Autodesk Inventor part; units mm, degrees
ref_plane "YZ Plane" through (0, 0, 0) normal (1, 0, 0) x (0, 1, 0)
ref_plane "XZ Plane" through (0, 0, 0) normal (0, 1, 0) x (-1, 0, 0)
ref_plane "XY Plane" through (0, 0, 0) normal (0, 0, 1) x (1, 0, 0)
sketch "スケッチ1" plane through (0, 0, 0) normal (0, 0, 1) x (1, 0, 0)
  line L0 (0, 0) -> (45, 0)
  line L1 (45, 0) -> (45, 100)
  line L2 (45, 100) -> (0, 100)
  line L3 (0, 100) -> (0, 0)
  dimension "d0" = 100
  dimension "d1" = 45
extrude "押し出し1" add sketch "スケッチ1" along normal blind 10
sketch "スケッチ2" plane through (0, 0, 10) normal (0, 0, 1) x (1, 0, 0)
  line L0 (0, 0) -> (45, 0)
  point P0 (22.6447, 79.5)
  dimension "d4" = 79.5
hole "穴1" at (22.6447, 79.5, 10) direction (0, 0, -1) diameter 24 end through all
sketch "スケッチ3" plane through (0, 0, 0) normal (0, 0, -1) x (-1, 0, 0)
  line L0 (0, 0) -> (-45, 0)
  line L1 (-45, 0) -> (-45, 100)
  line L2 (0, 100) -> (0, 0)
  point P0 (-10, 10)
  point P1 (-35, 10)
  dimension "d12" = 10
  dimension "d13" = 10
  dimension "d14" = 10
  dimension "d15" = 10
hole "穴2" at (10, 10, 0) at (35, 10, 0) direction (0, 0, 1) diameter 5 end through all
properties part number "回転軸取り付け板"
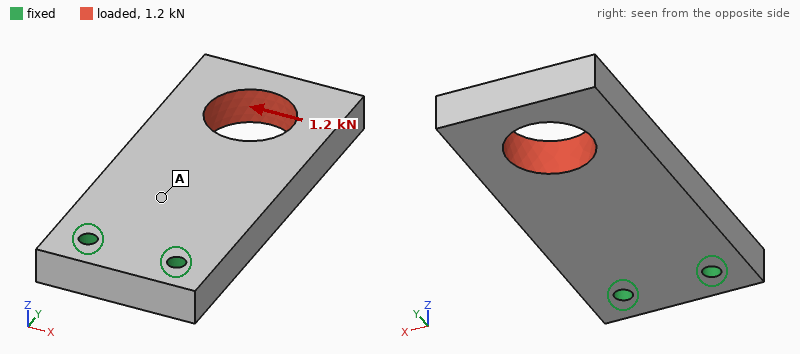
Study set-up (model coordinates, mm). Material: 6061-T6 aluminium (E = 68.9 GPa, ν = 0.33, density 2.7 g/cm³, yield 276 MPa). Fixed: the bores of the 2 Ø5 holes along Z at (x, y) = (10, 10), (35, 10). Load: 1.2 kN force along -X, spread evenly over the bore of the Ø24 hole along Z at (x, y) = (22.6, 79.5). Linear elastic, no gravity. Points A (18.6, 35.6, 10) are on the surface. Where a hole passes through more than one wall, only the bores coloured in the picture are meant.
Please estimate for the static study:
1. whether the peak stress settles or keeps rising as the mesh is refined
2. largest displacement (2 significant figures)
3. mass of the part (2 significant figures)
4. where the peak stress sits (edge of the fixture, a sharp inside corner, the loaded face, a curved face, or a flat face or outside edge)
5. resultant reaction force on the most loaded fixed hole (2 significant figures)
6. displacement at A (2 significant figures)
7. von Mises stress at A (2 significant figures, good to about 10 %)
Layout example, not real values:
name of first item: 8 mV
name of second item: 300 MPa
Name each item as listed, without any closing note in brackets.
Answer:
whether the peak stress settles or keeps rising as the mesh is refined: keeps rising
largest displacement: 63 µm
mass of the part: 110 g
where the peak stress sits: edge of the fixture
resultant reaction force on the most loaded fixed hole: 3.0 kN
displacement at A: 9.8 µm
von Mises stress at A: 7.9 MPa
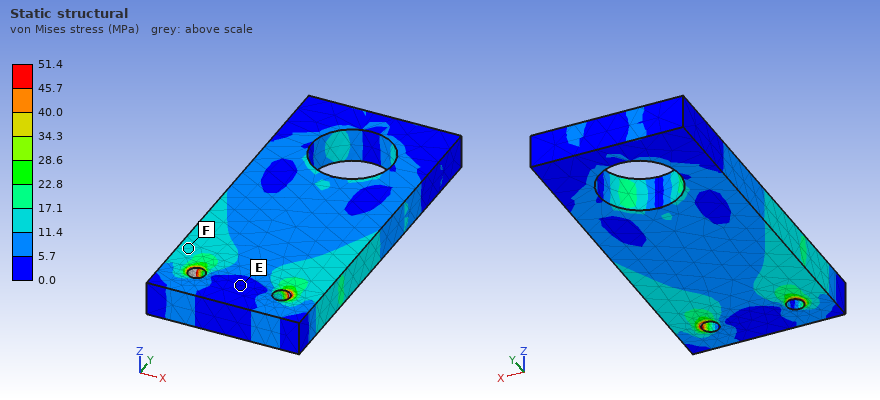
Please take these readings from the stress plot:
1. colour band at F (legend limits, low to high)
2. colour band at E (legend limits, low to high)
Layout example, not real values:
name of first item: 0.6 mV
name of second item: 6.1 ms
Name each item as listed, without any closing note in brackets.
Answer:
colour band at F: 11.4 to 17.1 MPa
colour band at E: 0.0 to 5.7 MPa
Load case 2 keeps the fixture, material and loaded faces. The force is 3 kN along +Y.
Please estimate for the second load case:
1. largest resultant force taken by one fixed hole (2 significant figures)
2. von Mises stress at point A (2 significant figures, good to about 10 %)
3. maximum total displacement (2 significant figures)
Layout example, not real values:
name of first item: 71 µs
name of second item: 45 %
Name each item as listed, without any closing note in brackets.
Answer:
largest resultant force taken by one fixed hole: 1.5 kN
von Mises stress at point A: 6.1 MPa
maximum total displacement: 14 µm
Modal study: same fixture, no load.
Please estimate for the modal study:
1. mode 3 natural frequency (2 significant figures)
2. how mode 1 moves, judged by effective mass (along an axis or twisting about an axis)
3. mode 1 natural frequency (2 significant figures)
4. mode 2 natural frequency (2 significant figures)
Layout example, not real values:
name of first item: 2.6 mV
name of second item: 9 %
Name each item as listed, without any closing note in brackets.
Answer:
mode 3 natural frequency: 3800 Hz
how mode 1 moves, judged by effective mass: along Z
mode 1 natural frequency: 1100 Hz
mode 2 natural frequency: 3700 Hz
